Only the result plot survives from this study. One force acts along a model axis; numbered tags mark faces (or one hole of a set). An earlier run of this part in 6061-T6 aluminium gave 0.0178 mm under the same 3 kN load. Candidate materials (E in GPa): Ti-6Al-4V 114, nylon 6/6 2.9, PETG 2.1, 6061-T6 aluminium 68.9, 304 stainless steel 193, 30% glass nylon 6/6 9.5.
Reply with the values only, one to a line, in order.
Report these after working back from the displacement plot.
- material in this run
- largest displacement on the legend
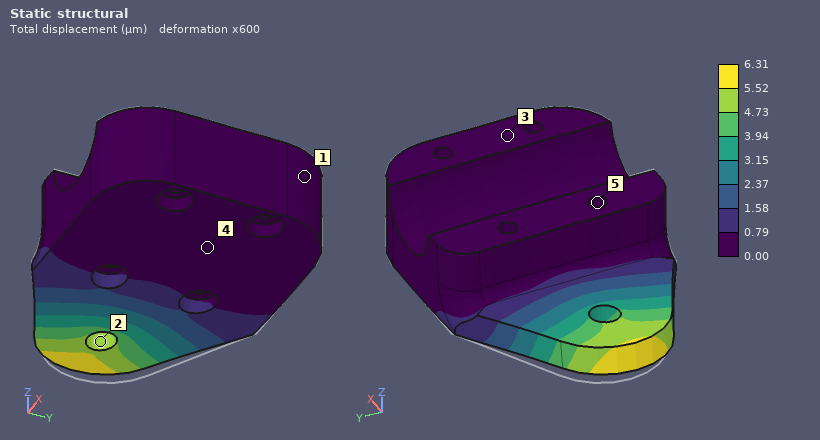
304 stainless steel
6.31 µm
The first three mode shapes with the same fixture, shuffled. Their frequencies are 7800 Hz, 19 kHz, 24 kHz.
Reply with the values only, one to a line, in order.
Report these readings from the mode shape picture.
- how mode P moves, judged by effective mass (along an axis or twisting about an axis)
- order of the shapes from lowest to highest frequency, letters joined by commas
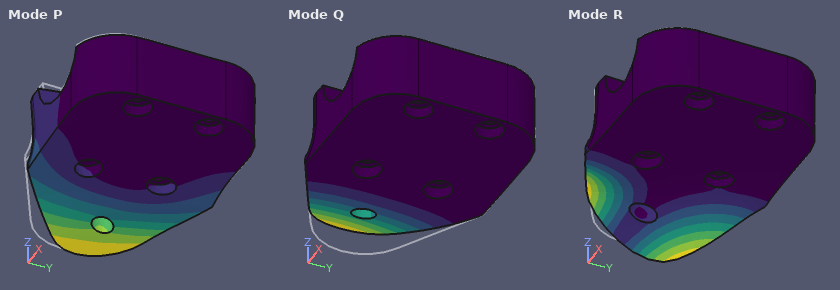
along Y
Q, R, P
